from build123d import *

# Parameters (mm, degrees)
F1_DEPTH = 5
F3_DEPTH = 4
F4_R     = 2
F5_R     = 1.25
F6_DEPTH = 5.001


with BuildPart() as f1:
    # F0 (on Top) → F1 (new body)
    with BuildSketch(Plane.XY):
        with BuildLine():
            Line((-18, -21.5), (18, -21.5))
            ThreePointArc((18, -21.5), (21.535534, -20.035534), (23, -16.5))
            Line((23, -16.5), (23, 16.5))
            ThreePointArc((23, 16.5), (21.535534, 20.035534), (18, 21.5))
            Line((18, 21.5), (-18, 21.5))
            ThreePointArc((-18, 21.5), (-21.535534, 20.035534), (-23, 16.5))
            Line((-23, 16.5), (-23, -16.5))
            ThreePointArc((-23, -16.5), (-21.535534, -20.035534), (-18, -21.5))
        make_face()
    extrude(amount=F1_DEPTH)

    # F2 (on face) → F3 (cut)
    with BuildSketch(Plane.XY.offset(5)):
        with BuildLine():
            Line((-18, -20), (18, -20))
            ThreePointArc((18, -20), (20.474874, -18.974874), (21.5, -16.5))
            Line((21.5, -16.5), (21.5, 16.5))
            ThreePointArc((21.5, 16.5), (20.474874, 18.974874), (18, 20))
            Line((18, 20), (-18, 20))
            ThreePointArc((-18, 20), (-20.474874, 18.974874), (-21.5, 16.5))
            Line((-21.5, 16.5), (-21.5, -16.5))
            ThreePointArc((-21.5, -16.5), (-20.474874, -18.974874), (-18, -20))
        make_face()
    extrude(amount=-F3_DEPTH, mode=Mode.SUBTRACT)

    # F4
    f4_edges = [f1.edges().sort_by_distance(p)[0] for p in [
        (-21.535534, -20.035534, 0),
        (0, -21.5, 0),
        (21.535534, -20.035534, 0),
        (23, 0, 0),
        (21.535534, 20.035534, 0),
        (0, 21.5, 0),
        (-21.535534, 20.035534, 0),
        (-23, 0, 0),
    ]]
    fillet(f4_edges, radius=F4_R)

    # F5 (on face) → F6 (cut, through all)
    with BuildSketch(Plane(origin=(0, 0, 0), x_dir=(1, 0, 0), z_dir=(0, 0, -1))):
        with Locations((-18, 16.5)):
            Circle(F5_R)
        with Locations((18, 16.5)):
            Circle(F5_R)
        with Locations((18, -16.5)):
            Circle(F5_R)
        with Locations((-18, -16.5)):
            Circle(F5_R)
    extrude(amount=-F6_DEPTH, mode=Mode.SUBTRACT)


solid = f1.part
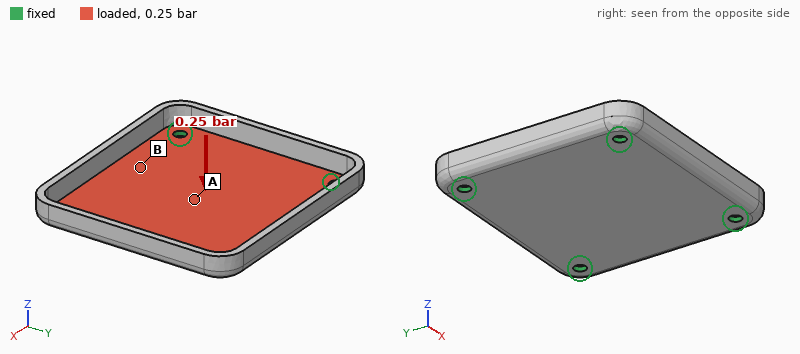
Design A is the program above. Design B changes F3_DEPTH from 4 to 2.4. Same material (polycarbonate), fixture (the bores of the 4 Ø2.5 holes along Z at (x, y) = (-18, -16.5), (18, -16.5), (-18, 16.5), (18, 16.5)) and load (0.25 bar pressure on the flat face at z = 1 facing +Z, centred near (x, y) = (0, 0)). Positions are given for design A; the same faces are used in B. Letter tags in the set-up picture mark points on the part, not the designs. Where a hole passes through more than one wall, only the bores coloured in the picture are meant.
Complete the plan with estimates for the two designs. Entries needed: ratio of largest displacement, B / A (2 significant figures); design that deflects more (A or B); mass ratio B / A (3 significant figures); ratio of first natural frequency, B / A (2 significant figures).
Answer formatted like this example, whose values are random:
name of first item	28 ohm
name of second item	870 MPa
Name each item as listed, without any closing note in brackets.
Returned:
ratio of largest displacement, B / A	0.084
design that deflects more	A
mass ratio B / A	1.97
ratio of first natural frequency, B / A	2.1
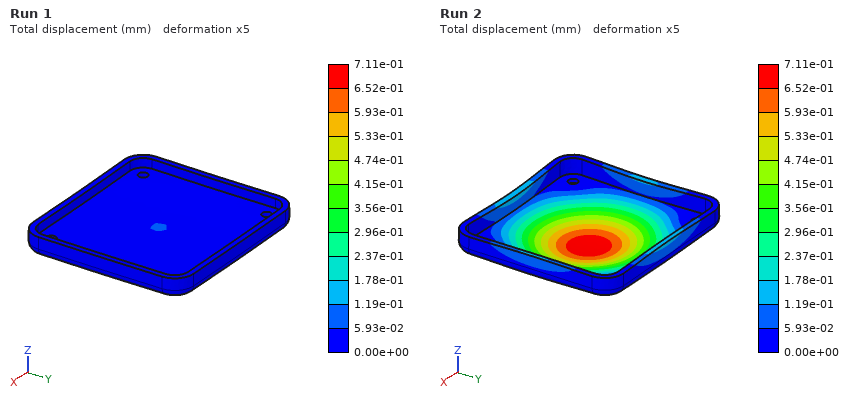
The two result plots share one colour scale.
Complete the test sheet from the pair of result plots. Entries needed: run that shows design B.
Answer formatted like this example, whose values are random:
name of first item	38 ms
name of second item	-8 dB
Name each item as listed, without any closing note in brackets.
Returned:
run that shows design B	Run 1
